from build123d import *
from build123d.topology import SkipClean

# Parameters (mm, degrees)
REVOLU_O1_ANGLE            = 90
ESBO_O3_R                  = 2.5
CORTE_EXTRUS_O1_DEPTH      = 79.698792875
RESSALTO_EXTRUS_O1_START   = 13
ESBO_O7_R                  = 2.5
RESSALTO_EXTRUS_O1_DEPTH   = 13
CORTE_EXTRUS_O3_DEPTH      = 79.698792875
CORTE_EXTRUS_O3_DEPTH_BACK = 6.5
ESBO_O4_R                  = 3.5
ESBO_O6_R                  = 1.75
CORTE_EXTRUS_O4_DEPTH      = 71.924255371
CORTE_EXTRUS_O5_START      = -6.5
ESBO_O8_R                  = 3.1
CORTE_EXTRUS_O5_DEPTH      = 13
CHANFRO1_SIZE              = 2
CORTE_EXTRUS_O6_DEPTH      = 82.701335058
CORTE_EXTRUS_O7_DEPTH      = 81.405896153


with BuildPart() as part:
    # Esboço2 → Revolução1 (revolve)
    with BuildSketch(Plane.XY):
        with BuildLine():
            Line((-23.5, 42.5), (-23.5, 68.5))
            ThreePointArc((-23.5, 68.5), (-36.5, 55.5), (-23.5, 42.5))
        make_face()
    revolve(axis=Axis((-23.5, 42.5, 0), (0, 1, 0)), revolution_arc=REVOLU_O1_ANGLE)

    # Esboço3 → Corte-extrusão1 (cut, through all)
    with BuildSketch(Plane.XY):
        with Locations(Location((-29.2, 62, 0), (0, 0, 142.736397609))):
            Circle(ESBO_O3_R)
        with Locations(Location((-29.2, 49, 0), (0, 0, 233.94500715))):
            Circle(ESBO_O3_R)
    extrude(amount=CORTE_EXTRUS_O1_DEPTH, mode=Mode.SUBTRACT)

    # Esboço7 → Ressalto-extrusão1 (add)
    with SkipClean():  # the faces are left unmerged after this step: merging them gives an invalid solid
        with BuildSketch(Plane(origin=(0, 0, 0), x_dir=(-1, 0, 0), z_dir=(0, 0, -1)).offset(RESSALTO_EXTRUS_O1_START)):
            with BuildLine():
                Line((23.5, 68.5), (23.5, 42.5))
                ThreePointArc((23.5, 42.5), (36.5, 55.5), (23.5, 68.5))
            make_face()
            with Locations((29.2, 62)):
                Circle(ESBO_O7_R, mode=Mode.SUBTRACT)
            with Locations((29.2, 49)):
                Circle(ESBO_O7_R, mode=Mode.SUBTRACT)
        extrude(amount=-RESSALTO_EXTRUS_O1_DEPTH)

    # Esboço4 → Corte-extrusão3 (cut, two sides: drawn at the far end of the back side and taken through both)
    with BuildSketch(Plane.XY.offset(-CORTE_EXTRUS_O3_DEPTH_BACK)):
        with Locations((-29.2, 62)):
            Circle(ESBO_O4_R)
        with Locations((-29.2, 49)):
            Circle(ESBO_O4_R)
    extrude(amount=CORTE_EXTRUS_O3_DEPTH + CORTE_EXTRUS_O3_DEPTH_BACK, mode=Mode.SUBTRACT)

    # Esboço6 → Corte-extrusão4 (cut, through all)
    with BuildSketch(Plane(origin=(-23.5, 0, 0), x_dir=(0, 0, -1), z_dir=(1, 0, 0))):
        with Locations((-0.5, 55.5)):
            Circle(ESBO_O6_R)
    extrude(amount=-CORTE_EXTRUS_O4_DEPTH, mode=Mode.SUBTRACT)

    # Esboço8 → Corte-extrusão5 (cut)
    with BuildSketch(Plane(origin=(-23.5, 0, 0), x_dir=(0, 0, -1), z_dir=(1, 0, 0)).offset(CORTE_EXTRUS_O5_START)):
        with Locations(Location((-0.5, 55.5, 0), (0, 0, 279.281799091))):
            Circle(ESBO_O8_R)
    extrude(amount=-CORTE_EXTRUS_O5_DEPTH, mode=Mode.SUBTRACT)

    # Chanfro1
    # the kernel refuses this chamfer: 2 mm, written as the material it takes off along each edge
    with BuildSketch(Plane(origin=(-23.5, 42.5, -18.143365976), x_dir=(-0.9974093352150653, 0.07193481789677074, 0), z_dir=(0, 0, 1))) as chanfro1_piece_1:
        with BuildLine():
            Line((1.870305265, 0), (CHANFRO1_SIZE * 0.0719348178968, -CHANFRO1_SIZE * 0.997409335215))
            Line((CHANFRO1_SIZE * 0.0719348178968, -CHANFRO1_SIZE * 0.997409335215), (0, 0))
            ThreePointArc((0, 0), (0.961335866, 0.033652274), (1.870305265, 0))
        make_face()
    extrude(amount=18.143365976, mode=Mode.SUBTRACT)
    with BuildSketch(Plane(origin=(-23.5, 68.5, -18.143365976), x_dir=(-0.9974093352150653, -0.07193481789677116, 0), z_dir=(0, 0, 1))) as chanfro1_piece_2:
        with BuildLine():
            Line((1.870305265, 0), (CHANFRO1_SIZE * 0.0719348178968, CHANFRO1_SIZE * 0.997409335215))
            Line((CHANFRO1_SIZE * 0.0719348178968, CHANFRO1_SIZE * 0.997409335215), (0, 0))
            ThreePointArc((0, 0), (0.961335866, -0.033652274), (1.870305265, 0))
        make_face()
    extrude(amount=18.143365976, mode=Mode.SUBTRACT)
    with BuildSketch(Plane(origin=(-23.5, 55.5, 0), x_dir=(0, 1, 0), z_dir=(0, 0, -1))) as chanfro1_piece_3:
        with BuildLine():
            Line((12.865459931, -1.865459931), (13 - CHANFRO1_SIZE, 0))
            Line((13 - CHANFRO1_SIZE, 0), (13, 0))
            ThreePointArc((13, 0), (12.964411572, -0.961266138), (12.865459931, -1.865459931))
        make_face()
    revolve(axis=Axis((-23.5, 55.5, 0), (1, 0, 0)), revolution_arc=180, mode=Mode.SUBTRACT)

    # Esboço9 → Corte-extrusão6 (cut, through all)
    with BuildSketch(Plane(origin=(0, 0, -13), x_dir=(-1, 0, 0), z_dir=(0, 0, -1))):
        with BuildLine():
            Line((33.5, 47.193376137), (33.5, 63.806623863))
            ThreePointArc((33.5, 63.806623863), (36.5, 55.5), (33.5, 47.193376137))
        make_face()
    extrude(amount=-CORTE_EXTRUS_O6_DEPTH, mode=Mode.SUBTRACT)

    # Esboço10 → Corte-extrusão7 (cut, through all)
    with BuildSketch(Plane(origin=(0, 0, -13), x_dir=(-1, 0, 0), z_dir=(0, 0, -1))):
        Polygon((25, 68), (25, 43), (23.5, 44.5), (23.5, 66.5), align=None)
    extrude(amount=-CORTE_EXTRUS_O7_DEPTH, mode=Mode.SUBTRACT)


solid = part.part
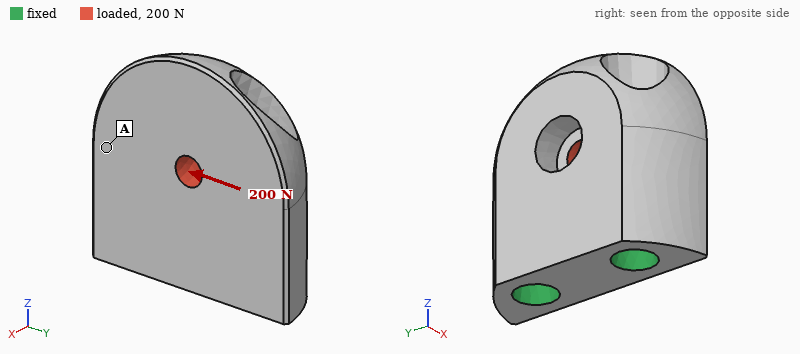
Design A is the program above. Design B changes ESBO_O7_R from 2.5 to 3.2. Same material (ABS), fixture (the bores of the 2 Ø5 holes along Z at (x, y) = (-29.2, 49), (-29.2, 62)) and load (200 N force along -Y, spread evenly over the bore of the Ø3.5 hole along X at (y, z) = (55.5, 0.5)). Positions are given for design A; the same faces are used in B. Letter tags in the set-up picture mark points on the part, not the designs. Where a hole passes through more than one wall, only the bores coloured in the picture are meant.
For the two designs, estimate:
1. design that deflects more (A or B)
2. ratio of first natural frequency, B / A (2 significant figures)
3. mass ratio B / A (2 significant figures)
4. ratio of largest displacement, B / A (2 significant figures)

A
1.1
0.94
0.92
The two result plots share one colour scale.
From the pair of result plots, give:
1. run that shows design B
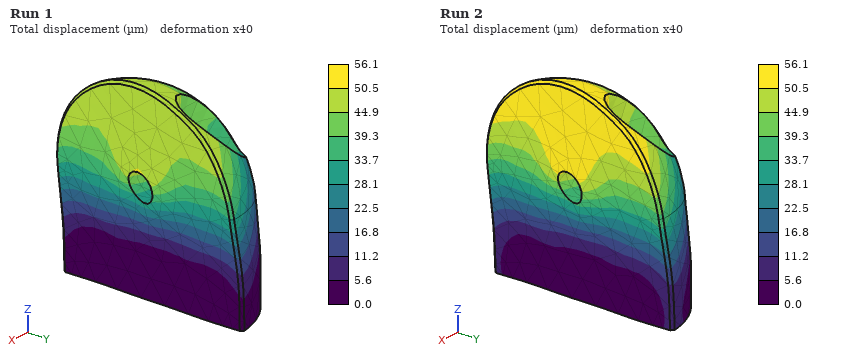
Run 1
